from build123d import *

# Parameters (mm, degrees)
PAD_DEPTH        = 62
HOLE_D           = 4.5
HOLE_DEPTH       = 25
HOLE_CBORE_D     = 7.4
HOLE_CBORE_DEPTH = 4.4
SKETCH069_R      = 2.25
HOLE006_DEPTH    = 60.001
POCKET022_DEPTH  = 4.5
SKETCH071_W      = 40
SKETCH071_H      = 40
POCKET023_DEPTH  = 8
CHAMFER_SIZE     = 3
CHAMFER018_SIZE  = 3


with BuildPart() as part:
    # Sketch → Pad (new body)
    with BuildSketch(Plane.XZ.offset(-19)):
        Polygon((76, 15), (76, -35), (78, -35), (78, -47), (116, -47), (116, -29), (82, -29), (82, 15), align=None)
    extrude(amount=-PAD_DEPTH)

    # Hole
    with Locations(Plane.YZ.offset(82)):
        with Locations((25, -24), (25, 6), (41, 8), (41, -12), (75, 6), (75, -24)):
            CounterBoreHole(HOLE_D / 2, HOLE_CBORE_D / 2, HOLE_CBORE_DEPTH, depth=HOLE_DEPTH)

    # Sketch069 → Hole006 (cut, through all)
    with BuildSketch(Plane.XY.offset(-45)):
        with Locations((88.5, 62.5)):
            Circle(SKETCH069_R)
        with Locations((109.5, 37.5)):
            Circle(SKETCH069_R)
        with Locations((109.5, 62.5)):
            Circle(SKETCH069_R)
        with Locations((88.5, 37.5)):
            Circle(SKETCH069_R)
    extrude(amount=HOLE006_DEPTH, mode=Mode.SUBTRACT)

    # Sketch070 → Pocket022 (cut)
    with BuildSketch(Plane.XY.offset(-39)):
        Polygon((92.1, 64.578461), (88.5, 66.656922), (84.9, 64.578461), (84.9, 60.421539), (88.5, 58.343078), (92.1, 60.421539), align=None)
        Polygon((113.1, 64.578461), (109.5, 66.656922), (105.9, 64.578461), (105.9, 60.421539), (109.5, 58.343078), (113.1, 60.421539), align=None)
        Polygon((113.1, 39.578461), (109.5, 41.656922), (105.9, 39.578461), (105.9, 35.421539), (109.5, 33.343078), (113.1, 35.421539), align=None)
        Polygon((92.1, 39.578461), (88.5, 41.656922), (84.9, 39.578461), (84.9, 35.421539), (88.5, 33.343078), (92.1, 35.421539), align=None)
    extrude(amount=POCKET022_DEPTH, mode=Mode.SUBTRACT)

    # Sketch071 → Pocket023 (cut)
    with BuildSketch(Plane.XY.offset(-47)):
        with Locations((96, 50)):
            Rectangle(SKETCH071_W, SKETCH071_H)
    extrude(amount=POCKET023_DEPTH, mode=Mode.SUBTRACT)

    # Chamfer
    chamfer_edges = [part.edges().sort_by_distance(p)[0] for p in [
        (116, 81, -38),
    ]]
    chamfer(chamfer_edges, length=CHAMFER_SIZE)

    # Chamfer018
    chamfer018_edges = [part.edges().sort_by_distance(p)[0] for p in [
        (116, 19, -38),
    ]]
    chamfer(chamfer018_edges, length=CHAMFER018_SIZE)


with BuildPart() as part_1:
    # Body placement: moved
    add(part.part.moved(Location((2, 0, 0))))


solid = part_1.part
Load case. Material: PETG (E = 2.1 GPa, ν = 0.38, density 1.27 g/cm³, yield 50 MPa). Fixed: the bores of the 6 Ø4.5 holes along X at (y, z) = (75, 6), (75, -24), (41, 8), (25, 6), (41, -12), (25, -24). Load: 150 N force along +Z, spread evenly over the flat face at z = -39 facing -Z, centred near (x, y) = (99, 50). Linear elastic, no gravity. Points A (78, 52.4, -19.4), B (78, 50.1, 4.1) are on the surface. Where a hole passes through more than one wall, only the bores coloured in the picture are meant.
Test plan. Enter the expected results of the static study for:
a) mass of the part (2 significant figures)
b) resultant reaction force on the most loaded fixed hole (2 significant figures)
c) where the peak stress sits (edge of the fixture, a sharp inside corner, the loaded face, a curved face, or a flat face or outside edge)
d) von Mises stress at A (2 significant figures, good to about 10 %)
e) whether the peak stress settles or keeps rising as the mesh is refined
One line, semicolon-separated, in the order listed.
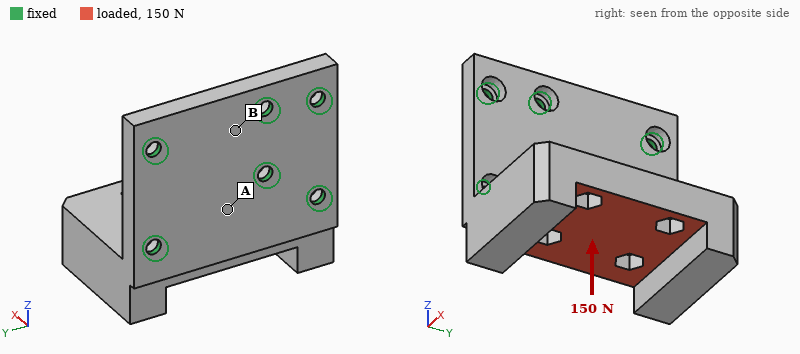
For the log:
57 g; 100 N; edge of the fixture; 3.1 MPa; keeps rising
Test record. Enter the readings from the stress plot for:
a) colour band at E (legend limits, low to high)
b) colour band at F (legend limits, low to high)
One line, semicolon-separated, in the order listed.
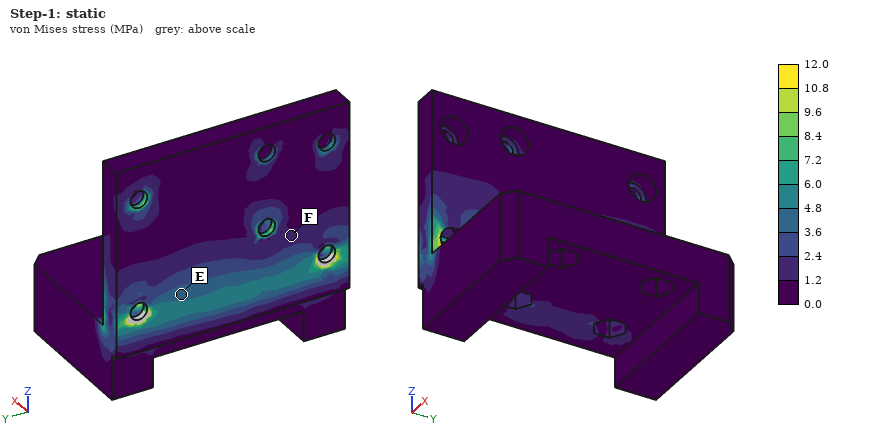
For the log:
3.6 to 4.8 MPa; 1.2 to 2.4 MPa
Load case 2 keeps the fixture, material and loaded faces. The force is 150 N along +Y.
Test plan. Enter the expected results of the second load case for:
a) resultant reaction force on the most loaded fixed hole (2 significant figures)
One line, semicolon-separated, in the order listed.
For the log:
94 N
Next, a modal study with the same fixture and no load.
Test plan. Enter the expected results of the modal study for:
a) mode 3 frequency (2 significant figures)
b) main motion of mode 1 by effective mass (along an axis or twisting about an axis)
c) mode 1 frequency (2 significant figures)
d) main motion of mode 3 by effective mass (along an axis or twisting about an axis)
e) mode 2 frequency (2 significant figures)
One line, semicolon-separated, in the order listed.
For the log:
1700 Hz; along Z; 440 Hz; along Y; 1100 Hz
